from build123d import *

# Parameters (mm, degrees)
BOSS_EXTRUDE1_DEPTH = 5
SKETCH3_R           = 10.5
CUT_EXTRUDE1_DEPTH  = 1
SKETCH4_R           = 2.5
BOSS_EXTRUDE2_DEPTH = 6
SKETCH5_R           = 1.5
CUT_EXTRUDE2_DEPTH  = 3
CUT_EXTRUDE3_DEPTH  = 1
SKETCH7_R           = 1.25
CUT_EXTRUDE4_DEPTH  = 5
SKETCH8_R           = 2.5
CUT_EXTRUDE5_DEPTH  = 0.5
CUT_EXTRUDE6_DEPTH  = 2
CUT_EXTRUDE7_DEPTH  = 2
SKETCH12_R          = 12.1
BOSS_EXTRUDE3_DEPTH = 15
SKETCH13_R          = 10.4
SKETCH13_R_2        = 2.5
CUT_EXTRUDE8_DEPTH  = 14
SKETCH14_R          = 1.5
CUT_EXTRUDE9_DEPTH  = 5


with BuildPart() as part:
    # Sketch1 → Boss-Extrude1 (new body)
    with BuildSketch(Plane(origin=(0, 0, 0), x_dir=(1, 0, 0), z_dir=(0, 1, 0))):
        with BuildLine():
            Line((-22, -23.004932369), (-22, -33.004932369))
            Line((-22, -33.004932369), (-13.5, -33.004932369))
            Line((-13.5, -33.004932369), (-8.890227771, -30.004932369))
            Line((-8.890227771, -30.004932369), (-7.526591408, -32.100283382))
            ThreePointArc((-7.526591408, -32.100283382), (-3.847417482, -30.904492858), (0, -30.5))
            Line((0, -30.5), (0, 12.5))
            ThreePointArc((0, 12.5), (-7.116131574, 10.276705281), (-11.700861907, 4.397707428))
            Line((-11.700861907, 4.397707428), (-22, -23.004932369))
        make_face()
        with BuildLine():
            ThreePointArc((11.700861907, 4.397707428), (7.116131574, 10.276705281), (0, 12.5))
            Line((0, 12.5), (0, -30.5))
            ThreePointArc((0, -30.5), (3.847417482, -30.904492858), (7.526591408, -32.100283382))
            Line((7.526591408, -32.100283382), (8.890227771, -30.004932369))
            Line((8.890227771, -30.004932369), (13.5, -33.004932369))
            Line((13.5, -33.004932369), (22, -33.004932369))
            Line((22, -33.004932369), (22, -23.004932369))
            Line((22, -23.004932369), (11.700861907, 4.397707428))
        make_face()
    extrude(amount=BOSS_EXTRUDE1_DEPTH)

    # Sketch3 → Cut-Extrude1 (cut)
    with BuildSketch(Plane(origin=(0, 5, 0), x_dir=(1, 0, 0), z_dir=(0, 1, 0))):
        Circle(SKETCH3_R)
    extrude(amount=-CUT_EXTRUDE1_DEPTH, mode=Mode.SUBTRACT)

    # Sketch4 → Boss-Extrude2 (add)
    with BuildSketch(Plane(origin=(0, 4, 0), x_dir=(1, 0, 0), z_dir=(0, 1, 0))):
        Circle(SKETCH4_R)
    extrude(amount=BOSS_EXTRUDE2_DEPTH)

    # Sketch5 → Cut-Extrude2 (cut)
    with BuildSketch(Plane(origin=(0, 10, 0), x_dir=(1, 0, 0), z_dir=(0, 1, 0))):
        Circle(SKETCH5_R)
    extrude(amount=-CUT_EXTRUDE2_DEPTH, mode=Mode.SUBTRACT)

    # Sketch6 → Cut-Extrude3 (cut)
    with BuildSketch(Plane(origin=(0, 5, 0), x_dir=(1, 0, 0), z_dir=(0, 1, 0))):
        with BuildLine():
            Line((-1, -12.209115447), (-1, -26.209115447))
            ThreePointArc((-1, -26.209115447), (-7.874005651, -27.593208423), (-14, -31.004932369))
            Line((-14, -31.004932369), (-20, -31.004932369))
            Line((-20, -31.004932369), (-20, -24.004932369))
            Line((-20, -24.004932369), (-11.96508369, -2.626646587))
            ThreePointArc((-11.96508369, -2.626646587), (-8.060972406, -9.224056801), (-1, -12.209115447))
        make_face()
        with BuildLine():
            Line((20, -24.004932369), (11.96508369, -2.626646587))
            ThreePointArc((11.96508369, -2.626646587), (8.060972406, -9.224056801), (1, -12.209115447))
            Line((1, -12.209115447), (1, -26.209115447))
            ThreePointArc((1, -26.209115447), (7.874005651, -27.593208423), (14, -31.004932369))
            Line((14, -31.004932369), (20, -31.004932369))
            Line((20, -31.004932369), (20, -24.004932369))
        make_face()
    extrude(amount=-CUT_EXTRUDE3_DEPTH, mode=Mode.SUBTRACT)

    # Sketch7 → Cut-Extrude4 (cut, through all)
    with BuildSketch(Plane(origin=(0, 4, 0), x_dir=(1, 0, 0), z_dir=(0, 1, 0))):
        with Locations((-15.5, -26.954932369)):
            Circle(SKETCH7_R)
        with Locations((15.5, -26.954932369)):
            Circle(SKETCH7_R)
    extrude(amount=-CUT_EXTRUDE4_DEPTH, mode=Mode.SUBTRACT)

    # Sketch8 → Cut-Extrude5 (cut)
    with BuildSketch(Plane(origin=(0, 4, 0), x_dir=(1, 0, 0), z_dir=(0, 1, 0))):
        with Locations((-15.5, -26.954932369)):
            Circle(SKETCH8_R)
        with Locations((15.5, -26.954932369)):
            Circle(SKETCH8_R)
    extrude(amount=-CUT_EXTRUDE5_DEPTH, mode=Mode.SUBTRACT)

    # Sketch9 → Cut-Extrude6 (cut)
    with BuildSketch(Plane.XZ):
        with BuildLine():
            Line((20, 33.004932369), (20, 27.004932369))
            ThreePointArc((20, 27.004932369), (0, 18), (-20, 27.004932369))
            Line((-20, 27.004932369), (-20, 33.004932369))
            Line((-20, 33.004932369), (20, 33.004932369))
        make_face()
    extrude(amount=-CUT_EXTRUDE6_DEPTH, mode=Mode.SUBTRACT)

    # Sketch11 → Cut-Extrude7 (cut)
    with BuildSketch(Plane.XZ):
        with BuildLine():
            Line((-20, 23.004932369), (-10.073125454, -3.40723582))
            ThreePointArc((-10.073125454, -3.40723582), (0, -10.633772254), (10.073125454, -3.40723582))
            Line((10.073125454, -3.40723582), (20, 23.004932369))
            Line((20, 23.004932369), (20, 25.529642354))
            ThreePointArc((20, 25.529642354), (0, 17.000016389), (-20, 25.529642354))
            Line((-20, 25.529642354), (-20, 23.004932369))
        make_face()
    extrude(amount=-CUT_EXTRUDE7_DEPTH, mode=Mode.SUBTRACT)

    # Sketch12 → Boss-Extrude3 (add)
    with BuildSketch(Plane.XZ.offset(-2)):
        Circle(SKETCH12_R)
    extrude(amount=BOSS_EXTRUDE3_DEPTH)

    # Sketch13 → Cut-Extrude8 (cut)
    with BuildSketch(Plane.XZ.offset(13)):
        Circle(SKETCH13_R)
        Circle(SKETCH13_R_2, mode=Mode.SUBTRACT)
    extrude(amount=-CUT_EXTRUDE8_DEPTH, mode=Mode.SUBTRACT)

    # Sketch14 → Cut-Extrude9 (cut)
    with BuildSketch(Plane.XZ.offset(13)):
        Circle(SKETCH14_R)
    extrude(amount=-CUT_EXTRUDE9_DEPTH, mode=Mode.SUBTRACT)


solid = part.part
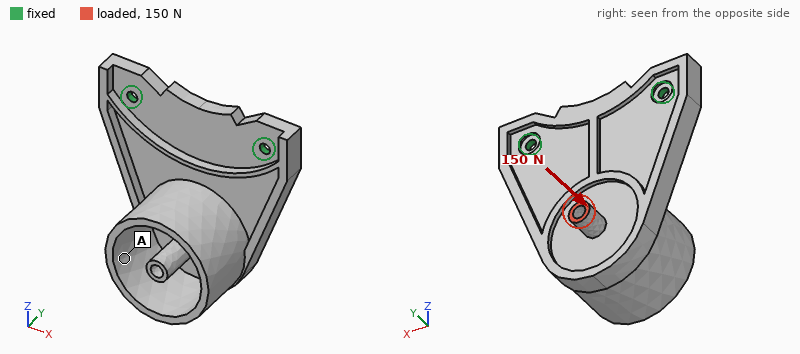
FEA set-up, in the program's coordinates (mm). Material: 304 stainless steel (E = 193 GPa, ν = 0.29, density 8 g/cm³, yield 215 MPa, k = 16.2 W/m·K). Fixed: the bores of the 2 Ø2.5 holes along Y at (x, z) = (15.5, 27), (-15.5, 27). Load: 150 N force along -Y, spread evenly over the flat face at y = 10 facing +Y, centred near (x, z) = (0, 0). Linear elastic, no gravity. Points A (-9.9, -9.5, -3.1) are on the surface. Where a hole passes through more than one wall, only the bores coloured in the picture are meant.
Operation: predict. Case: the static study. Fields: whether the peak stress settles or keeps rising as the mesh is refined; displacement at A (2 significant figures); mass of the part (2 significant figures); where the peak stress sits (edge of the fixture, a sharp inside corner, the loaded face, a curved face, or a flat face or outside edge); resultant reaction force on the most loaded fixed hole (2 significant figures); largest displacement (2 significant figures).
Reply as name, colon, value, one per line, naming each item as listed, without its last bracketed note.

whether the peak stress settles or keeps rising as the mesh is refined: keeps rising
displacement at A: 0.18 mm
mass of the part: 49 g
where the peak stress sits: edge of the fixture
resultant reaction force on the most loaded fixed hole: 78 N
largest displacement: 0.24 mm
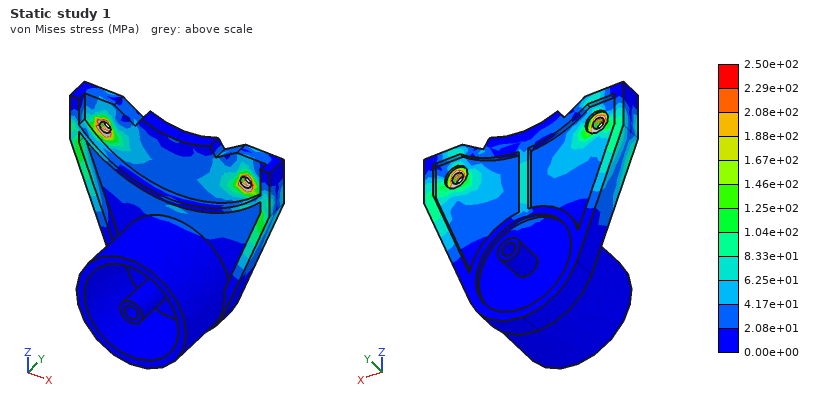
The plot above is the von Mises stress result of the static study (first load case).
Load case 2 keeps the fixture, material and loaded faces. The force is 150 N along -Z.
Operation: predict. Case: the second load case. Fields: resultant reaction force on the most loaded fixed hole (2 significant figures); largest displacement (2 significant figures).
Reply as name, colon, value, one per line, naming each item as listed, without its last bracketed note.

resultant reaction force on the most loaded fixed hole: 80 N
largest displacement: 84 µm
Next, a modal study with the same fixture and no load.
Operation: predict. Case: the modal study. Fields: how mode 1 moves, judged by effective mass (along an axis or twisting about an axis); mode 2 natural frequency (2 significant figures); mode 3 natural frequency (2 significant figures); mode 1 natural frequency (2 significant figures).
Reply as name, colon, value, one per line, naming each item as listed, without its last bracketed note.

how mode 1 moves, judged by effective mass: along Y
mode 2 natural frequency: 3300 Hz
mode 3 natural frequency: 5100 Hz
mode 1 natural frequency: 850 Hz
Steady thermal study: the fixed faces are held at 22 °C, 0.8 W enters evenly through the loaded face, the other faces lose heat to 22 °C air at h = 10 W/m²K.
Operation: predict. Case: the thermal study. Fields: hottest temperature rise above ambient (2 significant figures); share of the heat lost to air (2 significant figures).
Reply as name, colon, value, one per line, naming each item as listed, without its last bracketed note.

hottest temperature rise above ambient: 33 K
share of the heat lost to air: 52 %
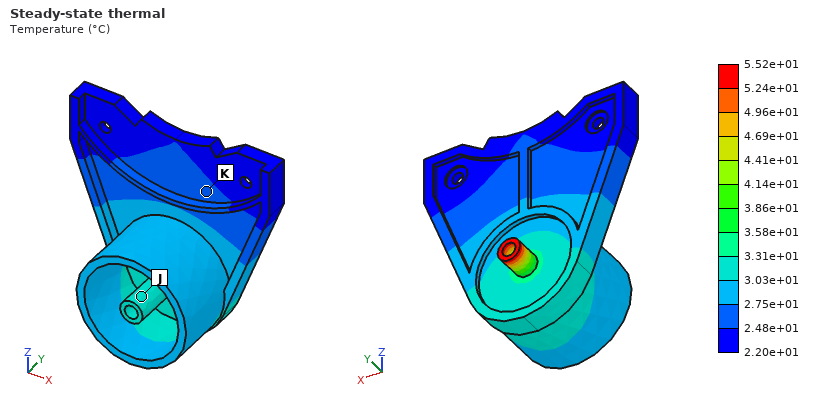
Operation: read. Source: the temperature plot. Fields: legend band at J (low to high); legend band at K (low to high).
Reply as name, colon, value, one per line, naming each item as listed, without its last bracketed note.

legend band at J: 3.03e+01 to 3.31e+01 °C
legend band at K: 2.48e+01 to 2.75e+01 °C
